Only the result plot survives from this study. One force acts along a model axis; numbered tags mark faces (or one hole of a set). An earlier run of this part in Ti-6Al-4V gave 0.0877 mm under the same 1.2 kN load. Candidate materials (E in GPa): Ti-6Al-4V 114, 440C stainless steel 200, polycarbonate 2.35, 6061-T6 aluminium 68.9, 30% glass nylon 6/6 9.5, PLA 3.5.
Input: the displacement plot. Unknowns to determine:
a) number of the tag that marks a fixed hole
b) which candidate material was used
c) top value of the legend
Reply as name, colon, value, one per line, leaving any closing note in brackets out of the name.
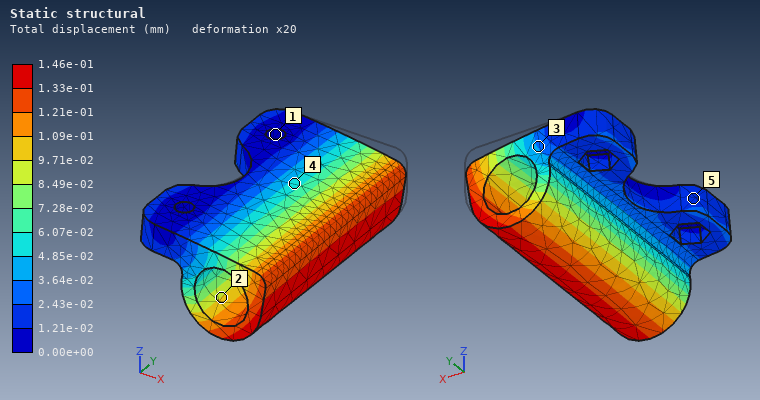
number of the tag that marks a fixed hole: 1
which candidate material was used: 6061-T6 aluminium
top value of the legend: 1.46e-01 mm
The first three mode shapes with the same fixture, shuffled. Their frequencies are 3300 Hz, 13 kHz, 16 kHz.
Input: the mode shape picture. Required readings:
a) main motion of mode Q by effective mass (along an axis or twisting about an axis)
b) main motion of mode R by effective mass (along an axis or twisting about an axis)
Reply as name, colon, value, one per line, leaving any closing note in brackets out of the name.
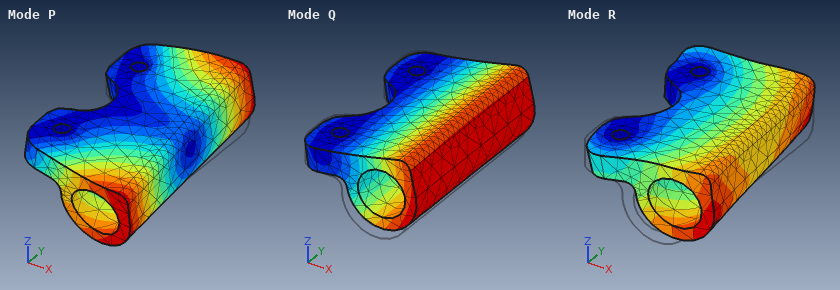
main motion of mode Q by effective mass: along Z
main motion of mode R by effective mass: along Y
